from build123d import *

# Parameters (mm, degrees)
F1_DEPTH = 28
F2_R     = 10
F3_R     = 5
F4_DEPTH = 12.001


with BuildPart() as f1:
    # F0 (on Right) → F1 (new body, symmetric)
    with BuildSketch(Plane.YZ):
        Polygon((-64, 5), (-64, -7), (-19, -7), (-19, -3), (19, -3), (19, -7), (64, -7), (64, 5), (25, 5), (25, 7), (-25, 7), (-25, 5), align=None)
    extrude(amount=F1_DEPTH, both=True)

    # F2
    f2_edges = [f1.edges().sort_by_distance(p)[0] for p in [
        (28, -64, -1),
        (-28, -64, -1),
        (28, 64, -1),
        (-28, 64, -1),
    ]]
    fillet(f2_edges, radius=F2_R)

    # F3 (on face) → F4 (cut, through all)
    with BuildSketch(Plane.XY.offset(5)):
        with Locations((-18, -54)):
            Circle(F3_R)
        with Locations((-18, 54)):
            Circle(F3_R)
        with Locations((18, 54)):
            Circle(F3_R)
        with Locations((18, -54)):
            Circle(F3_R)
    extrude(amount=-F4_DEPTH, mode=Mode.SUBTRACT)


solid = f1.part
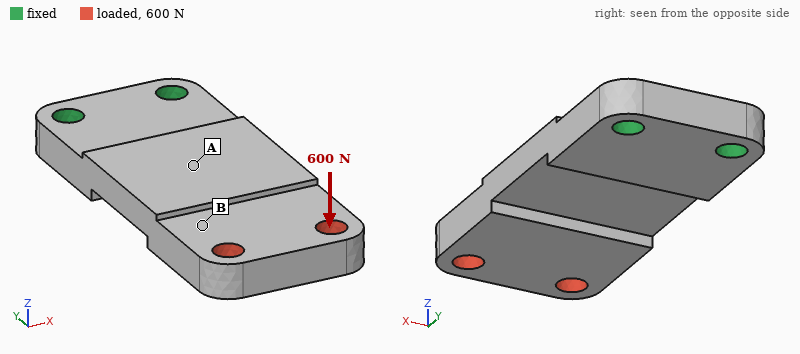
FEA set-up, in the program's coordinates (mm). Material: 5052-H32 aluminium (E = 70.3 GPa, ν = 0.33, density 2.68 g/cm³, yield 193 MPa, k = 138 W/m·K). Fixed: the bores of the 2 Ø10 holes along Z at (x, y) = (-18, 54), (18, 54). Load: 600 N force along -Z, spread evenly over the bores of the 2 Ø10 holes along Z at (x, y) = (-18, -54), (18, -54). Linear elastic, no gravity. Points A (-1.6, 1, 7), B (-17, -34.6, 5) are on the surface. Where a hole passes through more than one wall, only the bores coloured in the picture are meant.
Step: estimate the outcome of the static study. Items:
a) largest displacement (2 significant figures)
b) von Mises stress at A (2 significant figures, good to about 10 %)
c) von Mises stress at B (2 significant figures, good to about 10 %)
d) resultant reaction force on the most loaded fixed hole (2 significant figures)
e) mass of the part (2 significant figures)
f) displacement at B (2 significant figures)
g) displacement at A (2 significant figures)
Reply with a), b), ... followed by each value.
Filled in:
a) 0.60 mm
b) 33 MPa
c) 8.9 MPa
d) 300 N
e) 210 g
f) 0.37 mm
g) 0.14 mm
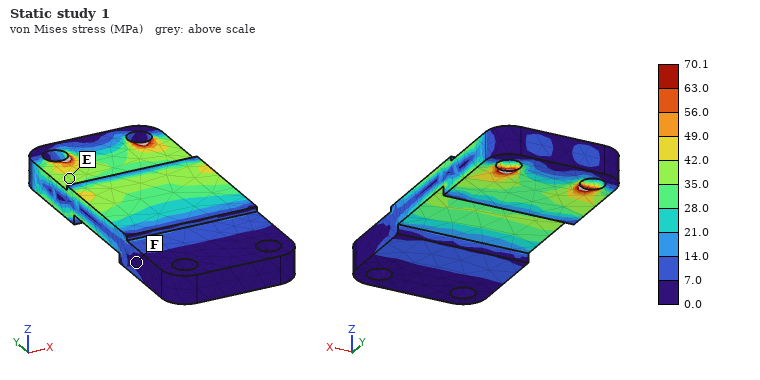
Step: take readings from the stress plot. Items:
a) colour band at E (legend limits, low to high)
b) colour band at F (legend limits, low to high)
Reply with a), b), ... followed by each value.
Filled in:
a) 35.0 to 42.0 MPa
b) 0.0 to 7.0 MPa
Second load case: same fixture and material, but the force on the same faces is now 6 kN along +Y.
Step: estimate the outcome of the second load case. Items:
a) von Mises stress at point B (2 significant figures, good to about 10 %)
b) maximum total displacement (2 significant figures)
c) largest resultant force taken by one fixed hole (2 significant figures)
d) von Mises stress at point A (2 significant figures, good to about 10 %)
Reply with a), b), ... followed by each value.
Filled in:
a) 8.6 MPa
b) 0.15 mm
c) 3.0 kN
d) 7.0 MPa
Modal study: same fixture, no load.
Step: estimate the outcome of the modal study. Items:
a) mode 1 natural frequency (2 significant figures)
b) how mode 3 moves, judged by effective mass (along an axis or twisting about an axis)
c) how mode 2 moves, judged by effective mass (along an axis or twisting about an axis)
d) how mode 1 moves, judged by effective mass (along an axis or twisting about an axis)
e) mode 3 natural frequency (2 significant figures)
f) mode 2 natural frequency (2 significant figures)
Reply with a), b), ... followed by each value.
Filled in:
a) 710 Hz
b) along X
c) along X
d) along Z
e) 3200 Hz
f) 2600 Hz
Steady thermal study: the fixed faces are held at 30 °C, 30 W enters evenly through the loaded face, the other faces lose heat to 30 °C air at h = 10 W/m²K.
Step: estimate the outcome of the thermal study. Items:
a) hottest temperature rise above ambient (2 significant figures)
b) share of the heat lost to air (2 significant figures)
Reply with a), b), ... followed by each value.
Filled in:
a) 37 K
b) 10 %
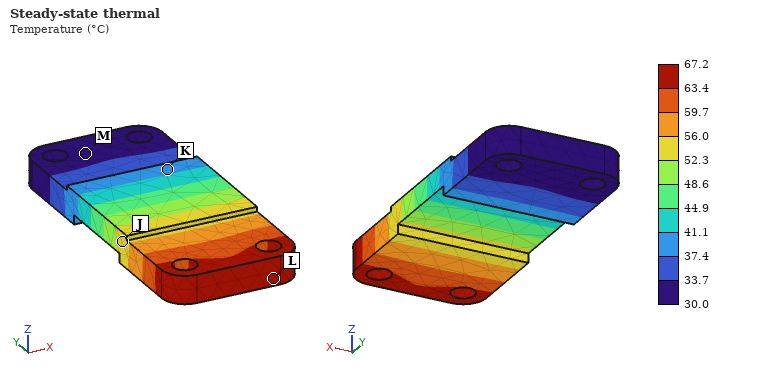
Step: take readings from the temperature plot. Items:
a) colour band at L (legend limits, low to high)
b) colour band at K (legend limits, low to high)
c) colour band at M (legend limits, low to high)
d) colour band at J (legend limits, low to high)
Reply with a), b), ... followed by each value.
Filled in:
a) 63.4 to 67.2 °C
b) 37.4 to 41.1 °C
c) 30.0 to 33.7 °C
d) 52.3 to 56.0 °C
